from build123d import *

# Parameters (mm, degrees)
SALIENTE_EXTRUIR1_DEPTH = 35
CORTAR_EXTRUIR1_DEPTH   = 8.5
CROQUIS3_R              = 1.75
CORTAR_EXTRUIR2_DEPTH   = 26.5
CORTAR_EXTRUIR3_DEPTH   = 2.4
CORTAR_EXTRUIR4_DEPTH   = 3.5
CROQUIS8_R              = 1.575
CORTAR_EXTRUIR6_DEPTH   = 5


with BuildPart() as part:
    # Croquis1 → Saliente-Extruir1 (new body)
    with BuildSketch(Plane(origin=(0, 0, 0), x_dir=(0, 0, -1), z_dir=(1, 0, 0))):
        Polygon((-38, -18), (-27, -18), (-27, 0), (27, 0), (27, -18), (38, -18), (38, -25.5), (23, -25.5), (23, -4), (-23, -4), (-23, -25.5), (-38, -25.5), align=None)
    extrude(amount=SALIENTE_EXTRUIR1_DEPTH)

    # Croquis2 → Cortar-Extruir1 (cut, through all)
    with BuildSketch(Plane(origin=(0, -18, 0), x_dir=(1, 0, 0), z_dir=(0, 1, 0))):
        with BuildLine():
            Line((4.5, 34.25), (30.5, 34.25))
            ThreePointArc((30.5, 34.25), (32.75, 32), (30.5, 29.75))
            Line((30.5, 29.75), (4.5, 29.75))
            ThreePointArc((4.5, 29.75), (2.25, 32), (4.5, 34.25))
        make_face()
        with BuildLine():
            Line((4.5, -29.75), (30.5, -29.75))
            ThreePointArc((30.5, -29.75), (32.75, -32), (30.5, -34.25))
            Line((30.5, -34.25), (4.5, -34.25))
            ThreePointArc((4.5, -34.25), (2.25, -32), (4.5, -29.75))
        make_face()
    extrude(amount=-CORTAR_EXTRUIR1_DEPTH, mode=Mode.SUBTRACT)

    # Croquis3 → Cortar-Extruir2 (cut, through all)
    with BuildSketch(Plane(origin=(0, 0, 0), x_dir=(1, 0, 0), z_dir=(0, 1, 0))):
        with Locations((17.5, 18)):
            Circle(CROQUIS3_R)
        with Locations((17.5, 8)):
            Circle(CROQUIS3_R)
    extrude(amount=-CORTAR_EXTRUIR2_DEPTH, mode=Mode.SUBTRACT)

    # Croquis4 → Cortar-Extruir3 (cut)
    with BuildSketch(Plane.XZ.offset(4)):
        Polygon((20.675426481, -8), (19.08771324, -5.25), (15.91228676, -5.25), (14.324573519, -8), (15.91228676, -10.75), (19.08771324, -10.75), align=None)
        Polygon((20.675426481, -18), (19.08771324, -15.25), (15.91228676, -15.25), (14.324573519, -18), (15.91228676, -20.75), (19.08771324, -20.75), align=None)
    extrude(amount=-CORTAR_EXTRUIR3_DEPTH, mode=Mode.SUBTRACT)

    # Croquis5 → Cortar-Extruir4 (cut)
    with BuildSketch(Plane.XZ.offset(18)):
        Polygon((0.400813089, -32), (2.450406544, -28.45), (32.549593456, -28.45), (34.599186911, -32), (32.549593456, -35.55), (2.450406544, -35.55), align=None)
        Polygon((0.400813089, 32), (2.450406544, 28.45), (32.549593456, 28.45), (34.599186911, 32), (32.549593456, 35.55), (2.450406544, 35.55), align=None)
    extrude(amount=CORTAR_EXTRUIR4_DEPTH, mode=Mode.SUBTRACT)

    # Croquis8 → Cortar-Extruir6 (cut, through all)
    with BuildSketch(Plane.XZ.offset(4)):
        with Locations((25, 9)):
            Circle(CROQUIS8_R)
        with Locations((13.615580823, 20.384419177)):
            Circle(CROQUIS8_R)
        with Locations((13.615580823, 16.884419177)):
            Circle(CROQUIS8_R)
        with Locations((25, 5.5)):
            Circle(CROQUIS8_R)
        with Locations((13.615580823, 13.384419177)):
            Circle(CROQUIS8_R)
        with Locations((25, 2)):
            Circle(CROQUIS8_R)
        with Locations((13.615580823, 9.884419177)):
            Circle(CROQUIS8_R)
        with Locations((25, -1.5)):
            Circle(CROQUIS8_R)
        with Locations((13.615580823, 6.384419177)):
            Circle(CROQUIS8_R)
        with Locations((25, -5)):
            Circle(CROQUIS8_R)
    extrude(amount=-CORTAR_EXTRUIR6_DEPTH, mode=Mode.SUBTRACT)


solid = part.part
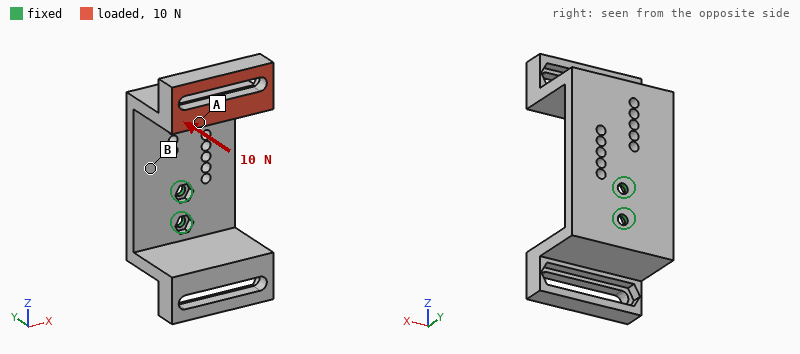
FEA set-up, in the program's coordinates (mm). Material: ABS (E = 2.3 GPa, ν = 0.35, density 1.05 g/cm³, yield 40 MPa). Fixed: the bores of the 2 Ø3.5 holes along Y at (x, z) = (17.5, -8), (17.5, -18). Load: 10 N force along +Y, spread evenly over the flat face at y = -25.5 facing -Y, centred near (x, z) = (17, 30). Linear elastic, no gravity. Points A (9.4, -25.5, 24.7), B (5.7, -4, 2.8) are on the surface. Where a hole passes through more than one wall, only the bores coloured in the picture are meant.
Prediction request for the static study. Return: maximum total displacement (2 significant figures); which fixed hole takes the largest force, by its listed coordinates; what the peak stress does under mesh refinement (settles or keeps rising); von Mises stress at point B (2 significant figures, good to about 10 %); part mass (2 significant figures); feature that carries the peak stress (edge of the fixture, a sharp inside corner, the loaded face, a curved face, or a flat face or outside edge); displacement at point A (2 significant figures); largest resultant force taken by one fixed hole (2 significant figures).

0.99 mm
(17.5, -8)
keeps rising
3.1 MPa
17 g
edge of the fixture
0.73 mm
44 N
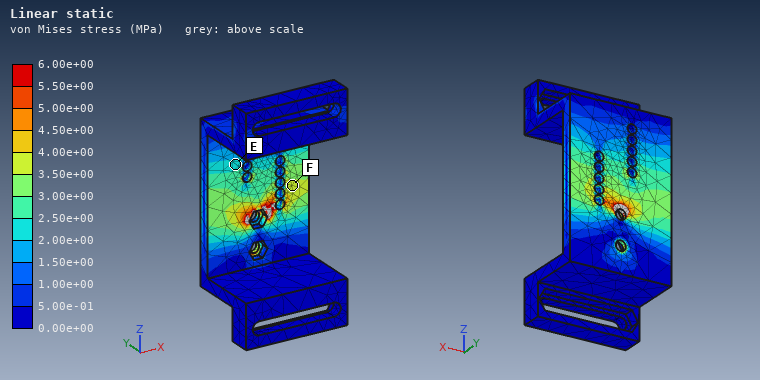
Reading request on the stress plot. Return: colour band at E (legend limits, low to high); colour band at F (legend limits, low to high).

2.00e+00 to 2.50e+00 MPa
3.50e+00 to 4.00e+00 MPa
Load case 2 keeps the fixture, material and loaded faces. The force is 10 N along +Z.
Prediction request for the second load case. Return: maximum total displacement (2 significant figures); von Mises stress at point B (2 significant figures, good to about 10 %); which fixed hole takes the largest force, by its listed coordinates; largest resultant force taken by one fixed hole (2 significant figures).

0.97 mm
2.8 MPa
(17.5, -18)
25 N
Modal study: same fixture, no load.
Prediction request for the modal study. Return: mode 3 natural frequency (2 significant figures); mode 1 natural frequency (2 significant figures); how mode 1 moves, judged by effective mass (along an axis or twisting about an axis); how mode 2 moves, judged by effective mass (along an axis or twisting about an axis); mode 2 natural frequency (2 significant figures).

620 Hz
240 Hz
along Y
along X
360 Hz
